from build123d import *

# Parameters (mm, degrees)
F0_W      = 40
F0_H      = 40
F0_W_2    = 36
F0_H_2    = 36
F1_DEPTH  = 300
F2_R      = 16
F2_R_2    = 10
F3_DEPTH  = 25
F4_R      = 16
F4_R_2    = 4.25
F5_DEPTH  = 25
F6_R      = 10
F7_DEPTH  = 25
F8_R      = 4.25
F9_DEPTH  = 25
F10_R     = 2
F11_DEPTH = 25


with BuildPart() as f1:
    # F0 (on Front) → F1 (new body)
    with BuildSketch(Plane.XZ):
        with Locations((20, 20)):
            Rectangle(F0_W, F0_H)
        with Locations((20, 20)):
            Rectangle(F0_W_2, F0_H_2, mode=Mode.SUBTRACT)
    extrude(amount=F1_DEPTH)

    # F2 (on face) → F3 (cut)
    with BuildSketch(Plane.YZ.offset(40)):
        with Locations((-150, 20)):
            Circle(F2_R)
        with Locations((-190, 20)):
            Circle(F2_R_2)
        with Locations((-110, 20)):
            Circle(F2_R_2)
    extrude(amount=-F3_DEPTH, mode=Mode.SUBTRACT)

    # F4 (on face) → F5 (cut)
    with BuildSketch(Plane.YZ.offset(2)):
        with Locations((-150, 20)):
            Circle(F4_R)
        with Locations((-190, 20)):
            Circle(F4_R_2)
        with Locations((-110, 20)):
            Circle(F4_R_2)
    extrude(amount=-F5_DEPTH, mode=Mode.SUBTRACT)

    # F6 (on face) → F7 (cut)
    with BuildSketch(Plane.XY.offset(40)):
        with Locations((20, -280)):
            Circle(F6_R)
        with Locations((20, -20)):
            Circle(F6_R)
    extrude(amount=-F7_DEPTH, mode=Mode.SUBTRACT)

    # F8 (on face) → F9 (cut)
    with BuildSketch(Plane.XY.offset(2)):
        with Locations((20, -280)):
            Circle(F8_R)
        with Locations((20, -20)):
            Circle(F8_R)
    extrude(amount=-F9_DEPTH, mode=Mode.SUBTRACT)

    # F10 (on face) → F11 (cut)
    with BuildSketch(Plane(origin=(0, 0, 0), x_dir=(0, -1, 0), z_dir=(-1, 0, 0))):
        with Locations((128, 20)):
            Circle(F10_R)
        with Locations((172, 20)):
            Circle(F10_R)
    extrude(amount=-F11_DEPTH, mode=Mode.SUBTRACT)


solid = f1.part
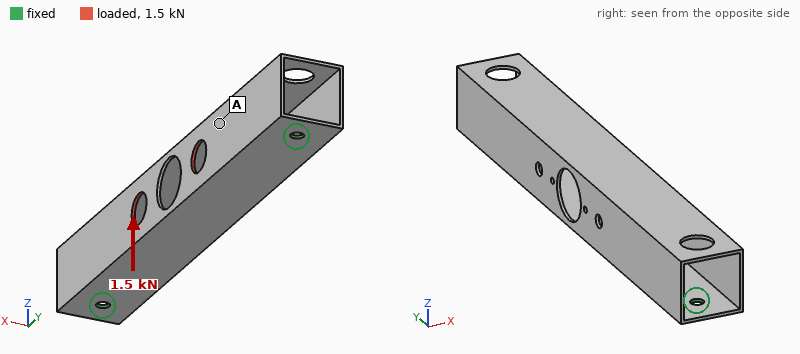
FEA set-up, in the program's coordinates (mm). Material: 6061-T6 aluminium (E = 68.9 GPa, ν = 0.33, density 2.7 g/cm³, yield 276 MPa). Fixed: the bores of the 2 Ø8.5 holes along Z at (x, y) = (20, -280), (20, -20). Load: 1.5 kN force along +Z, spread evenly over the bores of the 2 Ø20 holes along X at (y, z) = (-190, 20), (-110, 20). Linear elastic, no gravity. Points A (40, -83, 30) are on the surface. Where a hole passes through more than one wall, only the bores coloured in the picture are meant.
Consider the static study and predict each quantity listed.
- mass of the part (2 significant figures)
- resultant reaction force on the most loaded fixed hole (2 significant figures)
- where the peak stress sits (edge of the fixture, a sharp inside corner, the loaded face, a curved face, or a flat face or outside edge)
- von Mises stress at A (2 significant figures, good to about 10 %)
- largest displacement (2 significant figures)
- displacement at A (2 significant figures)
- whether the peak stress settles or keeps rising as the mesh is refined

230 g
1.3 kN
edge of the fixture
22 MPa
1.2 mm
0.99 mm
keeps rising
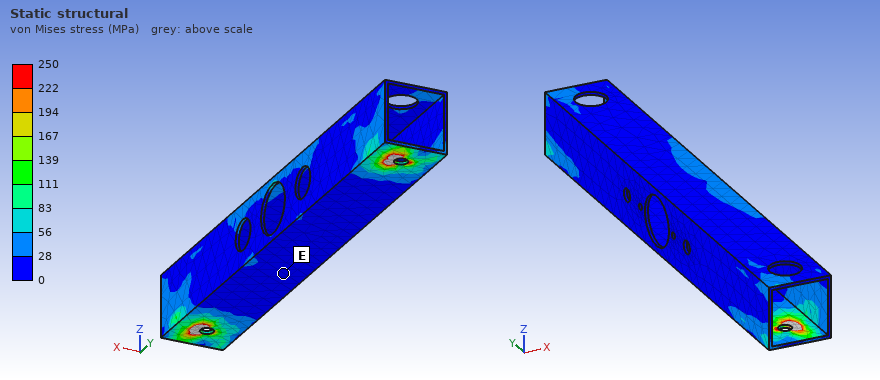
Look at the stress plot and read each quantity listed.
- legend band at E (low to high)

0 to 28 MPa
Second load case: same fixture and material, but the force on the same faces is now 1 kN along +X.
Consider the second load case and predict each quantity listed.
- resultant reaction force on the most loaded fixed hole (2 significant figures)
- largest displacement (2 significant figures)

500 N
0.94 mm
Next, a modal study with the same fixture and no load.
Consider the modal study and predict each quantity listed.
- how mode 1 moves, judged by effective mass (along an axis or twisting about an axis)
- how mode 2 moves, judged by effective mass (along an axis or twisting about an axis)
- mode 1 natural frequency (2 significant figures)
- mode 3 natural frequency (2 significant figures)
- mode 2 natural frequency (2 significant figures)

along X
along Z
370 Hz
1500 Hz
960 Hz
